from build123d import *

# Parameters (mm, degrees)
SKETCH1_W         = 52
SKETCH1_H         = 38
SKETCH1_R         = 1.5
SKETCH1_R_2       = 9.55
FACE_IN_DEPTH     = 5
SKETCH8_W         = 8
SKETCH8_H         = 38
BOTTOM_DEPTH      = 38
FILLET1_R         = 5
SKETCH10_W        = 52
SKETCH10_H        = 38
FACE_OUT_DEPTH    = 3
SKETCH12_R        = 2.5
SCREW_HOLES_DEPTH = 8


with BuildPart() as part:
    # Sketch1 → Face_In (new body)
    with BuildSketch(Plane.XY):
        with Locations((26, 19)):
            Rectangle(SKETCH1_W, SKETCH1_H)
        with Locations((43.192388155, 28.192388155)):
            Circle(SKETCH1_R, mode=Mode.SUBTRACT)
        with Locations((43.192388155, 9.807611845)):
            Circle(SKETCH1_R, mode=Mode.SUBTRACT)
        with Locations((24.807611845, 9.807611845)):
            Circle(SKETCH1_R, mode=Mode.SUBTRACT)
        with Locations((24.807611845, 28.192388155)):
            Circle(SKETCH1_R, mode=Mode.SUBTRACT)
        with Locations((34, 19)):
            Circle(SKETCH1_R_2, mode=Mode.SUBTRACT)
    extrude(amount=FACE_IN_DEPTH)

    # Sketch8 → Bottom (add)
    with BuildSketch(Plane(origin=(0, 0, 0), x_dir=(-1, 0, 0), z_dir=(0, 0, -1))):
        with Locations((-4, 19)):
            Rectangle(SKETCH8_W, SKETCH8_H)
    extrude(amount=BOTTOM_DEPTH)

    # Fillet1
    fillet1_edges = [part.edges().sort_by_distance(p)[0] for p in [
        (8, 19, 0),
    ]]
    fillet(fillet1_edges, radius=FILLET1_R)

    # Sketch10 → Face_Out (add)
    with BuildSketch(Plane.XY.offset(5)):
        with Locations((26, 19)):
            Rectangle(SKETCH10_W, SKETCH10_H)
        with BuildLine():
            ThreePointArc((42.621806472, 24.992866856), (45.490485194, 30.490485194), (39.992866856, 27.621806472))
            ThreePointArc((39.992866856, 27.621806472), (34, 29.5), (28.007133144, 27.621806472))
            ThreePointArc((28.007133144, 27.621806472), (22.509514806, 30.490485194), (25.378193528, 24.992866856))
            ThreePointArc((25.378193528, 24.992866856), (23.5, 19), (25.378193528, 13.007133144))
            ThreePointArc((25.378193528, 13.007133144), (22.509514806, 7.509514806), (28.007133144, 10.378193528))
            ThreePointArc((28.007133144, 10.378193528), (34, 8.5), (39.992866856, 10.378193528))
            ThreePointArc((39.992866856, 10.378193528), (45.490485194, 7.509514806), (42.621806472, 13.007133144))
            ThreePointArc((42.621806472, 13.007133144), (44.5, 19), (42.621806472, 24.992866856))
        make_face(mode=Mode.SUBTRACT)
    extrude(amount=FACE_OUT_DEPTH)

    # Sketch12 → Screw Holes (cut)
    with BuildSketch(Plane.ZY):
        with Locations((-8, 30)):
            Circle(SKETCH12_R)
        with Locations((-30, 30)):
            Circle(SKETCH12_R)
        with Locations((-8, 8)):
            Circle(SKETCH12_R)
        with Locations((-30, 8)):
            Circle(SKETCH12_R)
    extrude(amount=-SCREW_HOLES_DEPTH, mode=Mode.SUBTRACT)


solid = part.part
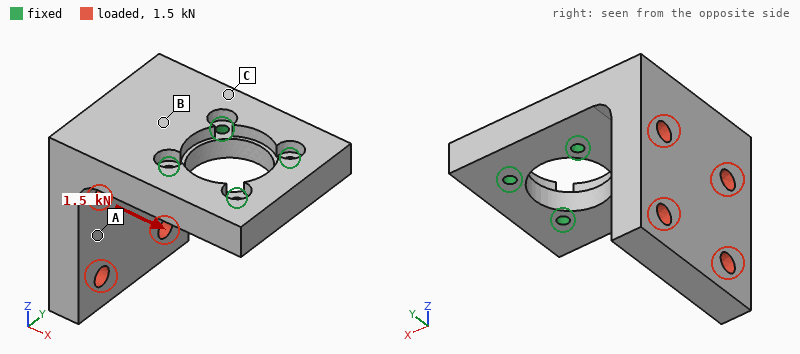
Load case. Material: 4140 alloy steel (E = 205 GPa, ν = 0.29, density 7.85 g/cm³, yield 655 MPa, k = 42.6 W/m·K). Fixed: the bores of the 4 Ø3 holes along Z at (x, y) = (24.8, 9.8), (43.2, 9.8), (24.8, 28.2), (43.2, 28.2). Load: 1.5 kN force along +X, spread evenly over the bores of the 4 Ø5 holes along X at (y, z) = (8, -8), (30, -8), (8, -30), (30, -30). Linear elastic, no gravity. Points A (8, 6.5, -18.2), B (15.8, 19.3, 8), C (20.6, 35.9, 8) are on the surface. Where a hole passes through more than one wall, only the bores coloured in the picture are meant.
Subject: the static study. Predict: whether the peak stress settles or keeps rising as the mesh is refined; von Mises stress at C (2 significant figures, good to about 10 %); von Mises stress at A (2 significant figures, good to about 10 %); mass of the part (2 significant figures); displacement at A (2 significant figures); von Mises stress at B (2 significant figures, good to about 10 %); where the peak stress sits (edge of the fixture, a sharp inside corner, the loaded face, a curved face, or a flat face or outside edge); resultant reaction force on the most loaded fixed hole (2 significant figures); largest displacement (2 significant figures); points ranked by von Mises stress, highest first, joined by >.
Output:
keeps rising
110 MPa
21 MPa
190 g
0.075 mm
58 MPa
edge of the fixture
1.2 kN
0.16 mm
C > B > A
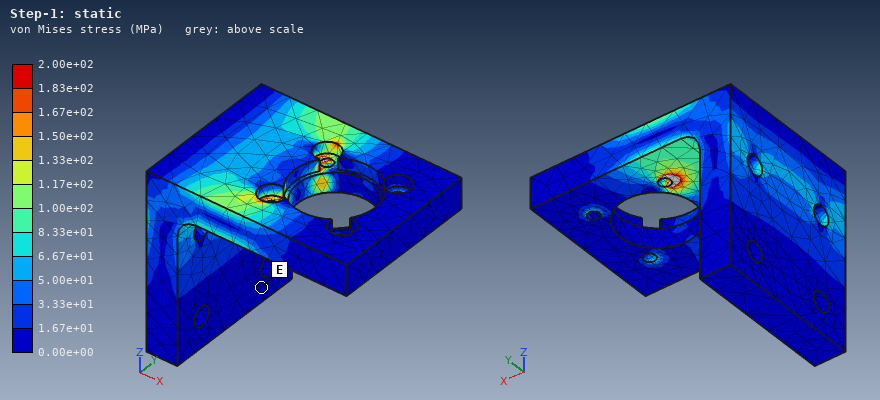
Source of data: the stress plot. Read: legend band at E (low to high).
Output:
0.00e+00 to 1.67e+01 MPa
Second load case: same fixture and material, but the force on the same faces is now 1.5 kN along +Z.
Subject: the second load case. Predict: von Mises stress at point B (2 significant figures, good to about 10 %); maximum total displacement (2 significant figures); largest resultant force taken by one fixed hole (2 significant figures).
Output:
27 MPa
86 µm
1.2 kN
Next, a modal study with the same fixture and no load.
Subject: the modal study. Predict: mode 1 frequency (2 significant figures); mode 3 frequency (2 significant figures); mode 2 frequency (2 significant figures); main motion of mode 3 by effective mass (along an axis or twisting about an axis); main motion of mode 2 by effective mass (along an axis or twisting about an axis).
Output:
1800 Hz
5900 Hz
3400 Hz
along Z
along Y
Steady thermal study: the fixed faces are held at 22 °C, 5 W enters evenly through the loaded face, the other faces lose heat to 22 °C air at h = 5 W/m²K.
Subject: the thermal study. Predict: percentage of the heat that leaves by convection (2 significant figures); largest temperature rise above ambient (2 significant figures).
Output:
6.6 %
17 K
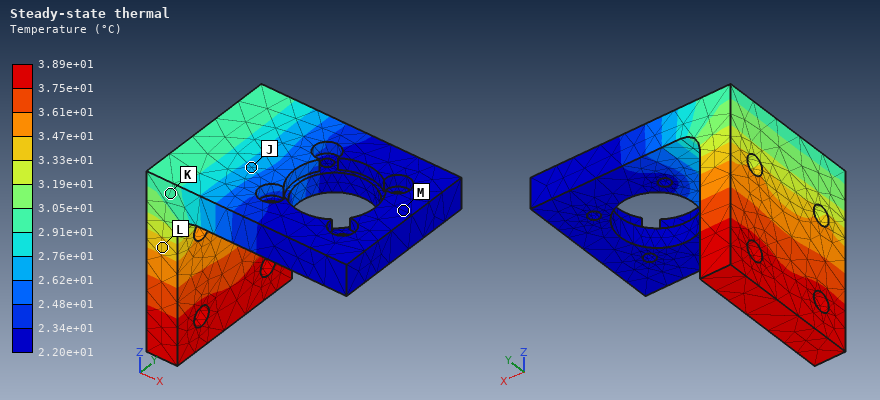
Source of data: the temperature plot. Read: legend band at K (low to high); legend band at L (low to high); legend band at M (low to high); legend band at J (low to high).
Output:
2.91e+01 to 3.05e+01 °C
3.33e+01 to 3.47e+01 °C
2.20e+01 to 2.34e+01 °C
2.62e+01 to 2.76e+01 °C
